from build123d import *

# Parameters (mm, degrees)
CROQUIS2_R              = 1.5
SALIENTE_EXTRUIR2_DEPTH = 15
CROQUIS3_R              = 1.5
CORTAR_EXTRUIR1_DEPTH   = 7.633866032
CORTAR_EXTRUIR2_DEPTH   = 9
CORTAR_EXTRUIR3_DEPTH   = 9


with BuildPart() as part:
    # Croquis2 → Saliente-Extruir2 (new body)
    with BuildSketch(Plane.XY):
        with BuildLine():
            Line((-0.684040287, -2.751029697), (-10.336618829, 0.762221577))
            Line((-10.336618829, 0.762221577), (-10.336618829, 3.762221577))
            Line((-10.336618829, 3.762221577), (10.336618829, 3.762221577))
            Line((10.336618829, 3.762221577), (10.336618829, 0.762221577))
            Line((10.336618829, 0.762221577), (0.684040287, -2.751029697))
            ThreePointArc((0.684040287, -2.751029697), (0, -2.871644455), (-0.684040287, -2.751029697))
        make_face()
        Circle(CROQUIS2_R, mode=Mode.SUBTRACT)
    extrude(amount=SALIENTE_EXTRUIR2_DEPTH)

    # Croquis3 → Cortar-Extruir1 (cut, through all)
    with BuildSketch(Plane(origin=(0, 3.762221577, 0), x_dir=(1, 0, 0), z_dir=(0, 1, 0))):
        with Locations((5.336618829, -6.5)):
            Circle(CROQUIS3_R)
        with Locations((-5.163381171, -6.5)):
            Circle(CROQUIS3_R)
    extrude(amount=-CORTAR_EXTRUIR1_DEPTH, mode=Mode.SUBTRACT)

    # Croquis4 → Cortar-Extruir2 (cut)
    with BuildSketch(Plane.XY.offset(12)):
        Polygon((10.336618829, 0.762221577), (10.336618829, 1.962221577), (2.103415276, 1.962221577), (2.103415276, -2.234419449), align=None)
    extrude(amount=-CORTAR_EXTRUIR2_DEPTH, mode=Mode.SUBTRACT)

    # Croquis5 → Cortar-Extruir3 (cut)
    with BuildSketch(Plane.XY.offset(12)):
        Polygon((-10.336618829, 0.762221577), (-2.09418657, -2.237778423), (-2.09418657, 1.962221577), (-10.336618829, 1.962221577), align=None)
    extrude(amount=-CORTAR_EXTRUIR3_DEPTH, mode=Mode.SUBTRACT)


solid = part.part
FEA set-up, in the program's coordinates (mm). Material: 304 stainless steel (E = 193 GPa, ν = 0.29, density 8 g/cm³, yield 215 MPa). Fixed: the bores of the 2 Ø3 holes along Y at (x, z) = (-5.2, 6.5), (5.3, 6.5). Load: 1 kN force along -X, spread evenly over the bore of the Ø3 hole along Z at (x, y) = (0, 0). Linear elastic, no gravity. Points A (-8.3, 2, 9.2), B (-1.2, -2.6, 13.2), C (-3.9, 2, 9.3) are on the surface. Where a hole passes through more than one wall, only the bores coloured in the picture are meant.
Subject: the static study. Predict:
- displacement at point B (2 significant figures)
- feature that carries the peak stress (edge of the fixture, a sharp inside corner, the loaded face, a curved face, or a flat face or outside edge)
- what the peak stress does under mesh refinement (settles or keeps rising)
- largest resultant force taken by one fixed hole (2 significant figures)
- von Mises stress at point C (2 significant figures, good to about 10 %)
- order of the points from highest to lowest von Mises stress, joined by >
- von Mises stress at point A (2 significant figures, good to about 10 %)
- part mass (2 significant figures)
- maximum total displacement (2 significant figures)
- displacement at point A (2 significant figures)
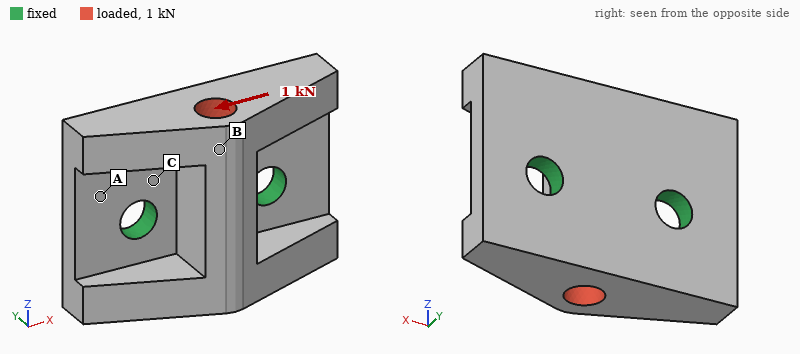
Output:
3.7 µm
edge of the fixture
keeps rising
580 N
41 MPa
C > A > B
23 MPa
7.8 g
5.4 µm
1.4 µm
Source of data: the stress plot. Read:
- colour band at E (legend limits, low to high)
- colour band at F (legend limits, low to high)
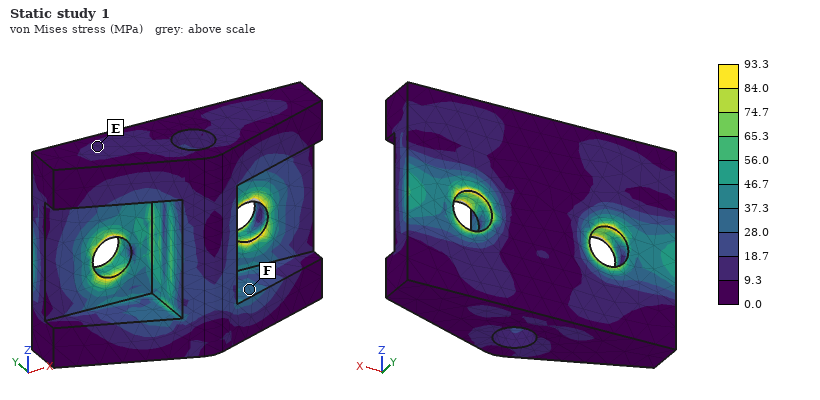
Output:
9.3 to 18.7 MPa
28.0 to 37.3 MPa
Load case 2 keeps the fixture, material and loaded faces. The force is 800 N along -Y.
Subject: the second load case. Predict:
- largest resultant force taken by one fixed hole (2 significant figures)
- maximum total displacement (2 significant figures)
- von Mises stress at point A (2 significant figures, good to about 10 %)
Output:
430 N
6.9 µm
28 MPa
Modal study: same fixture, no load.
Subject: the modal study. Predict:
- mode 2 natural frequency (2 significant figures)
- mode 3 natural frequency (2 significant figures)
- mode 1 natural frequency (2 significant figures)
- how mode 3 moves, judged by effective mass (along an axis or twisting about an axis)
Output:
28 kHz
36 kHz
17 kHz
along Y
